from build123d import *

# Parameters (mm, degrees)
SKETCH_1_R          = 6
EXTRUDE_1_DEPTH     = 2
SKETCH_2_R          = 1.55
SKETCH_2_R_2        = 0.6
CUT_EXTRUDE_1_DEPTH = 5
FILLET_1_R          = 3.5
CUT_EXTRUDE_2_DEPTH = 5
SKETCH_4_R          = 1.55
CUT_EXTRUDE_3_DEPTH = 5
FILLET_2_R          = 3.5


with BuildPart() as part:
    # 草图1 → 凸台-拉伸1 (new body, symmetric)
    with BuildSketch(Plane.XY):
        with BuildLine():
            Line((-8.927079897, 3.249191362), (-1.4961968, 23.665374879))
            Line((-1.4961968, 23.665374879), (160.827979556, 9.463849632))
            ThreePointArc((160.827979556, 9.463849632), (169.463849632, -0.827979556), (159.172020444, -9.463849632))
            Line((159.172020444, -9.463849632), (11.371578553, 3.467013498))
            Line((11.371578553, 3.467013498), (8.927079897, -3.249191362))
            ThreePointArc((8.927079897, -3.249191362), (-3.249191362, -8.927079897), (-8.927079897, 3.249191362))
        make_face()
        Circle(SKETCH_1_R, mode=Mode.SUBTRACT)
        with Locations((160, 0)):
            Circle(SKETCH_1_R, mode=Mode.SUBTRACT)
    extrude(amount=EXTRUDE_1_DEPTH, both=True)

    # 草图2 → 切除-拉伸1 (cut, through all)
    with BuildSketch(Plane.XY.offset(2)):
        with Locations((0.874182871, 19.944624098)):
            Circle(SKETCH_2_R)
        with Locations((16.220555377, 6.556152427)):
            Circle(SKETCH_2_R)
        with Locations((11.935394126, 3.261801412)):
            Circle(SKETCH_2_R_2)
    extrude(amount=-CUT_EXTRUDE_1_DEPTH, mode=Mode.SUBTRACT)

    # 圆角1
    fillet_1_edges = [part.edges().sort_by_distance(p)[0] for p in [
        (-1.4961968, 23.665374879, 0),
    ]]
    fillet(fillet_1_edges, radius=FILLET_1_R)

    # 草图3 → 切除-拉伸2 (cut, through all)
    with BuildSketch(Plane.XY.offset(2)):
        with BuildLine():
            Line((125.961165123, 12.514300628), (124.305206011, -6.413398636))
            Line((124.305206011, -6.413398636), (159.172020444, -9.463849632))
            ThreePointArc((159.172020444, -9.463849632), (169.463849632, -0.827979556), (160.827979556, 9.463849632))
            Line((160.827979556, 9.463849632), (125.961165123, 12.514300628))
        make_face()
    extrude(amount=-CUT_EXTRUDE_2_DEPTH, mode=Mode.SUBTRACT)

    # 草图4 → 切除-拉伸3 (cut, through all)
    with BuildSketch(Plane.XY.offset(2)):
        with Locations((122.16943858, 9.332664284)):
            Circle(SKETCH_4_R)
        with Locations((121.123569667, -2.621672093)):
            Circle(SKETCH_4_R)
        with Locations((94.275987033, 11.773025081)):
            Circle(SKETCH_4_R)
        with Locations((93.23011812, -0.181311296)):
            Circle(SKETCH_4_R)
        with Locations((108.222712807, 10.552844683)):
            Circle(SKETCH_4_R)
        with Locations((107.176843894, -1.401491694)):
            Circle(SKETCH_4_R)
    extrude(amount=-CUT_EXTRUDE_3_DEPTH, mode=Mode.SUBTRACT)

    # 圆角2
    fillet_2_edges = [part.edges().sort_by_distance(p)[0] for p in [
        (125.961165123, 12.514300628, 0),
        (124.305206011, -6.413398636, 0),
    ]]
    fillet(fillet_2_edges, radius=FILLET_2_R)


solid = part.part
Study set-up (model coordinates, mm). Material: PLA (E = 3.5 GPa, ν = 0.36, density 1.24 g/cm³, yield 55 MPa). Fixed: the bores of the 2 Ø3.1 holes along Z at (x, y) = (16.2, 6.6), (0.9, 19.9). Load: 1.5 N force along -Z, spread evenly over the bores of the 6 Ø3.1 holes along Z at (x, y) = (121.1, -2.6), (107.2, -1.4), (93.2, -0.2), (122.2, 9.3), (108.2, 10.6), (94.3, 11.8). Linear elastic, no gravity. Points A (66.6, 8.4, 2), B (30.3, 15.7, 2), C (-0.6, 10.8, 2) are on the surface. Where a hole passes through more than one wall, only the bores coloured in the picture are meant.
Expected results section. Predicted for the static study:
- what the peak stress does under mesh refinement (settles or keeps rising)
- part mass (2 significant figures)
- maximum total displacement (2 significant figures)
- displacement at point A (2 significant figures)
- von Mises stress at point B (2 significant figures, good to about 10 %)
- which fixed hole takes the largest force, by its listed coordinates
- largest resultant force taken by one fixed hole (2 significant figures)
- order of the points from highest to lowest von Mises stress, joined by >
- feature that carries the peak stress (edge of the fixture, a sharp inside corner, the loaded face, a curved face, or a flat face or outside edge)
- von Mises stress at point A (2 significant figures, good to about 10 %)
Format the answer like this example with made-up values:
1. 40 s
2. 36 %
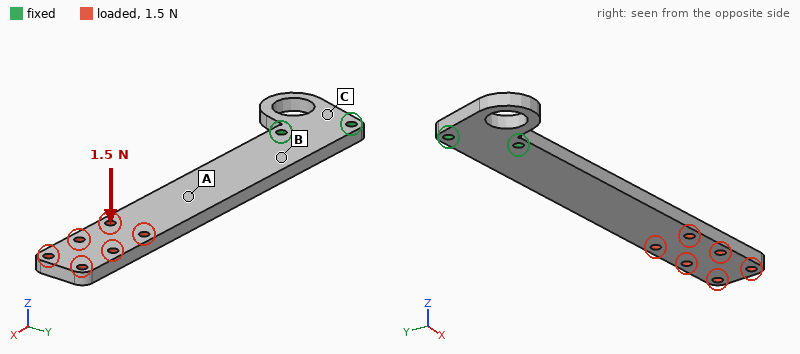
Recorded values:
1. keeps rising
2. 13 g
3. 1.4 mm
4. 0.42 mm
5. 2.2 MPa
6. (16.2, 6.6)
7. 5.1 N
8. B > A > C
9. edge of the fixture
10. 1.2 MPa
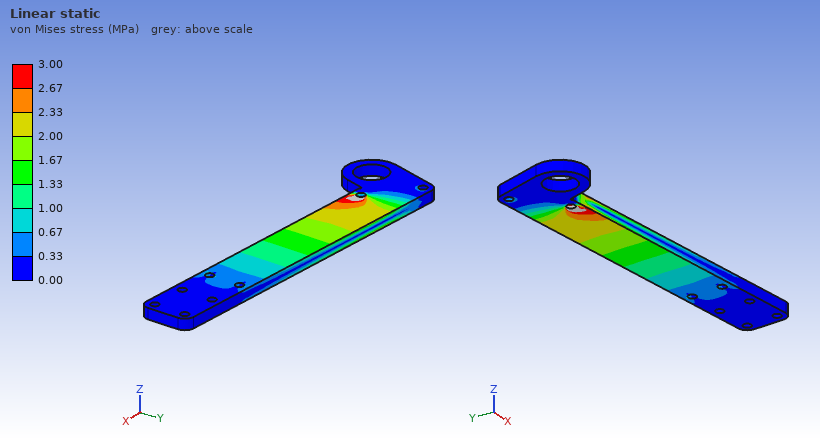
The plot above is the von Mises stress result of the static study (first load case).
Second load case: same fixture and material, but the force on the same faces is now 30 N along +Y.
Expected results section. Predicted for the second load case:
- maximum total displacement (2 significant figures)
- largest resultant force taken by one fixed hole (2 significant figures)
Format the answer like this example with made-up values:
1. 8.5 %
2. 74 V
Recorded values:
1. 1.5 mm
2. 160 N
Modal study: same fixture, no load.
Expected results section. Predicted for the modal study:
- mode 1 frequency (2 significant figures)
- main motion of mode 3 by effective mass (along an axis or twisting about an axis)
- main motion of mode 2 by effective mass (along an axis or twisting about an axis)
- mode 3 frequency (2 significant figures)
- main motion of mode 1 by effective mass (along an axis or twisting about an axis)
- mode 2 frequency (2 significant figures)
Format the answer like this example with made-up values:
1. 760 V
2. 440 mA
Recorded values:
1. 93 Hz
2. along Z
3. along Y
4. 560 Hz
5. along Z
6. 400 Hz
